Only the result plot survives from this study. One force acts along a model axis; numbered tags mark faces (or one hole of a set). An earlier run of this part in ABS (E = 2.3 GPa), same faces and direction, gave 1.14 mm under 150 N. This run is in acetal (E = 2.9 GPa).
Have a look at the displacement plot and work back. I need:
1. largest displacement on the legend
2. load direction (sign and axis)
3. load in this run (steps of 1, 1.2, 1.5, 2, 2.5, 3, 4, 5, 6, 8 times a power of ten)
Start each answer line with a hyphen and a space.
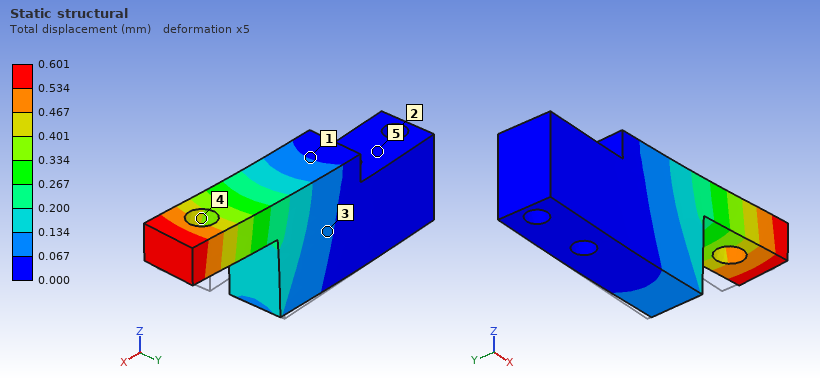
- 0.601 mm
- -Y
- 100 N
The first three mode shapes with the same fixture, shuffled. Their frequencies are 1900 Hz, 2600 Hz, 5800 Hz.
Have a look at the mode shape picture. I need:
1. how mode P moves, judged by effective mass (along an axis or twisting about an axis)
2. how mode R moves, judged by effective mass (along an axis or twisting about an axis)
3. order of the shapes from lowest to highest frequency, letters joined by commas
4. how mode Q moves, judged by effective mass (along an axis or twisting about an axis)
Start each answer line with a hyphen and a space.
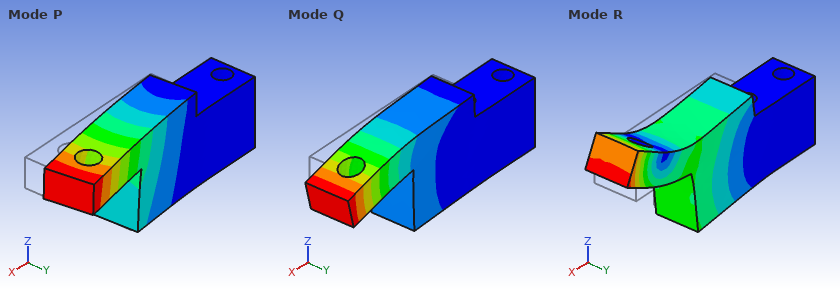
- along Y
- along Z
- P, Q, R
- along Z
